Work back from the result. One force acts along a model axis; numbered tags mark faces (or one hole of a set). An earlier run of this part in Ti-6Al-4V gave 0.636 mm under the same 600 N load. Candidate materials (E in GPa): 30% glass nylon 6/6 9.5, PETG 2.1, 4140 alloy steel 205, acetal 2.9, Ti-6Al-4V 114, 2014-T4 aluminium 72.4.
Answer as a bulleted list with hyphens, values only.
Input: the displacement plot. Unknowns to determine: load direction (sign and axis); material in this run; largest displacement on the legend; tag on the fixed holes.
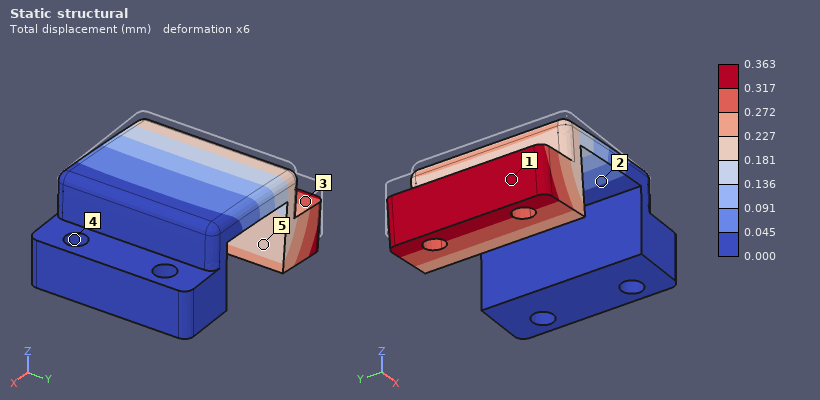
- -Z
- 4140 alloy steel
- 0.363 mm
- 4
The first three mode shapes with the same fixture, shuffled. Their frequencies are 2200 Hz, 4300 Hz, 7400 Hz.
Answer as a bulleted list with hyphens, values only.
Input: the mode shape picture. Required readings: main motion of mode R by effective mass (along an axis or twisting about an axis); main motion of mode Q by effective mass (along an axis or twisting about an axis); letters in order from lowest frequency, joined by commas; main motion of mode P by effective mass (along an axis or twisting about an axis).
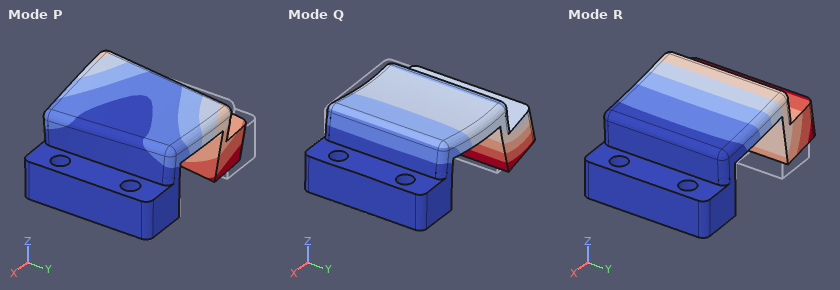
- along Z
- along X
- R, P, Q
- along Y
